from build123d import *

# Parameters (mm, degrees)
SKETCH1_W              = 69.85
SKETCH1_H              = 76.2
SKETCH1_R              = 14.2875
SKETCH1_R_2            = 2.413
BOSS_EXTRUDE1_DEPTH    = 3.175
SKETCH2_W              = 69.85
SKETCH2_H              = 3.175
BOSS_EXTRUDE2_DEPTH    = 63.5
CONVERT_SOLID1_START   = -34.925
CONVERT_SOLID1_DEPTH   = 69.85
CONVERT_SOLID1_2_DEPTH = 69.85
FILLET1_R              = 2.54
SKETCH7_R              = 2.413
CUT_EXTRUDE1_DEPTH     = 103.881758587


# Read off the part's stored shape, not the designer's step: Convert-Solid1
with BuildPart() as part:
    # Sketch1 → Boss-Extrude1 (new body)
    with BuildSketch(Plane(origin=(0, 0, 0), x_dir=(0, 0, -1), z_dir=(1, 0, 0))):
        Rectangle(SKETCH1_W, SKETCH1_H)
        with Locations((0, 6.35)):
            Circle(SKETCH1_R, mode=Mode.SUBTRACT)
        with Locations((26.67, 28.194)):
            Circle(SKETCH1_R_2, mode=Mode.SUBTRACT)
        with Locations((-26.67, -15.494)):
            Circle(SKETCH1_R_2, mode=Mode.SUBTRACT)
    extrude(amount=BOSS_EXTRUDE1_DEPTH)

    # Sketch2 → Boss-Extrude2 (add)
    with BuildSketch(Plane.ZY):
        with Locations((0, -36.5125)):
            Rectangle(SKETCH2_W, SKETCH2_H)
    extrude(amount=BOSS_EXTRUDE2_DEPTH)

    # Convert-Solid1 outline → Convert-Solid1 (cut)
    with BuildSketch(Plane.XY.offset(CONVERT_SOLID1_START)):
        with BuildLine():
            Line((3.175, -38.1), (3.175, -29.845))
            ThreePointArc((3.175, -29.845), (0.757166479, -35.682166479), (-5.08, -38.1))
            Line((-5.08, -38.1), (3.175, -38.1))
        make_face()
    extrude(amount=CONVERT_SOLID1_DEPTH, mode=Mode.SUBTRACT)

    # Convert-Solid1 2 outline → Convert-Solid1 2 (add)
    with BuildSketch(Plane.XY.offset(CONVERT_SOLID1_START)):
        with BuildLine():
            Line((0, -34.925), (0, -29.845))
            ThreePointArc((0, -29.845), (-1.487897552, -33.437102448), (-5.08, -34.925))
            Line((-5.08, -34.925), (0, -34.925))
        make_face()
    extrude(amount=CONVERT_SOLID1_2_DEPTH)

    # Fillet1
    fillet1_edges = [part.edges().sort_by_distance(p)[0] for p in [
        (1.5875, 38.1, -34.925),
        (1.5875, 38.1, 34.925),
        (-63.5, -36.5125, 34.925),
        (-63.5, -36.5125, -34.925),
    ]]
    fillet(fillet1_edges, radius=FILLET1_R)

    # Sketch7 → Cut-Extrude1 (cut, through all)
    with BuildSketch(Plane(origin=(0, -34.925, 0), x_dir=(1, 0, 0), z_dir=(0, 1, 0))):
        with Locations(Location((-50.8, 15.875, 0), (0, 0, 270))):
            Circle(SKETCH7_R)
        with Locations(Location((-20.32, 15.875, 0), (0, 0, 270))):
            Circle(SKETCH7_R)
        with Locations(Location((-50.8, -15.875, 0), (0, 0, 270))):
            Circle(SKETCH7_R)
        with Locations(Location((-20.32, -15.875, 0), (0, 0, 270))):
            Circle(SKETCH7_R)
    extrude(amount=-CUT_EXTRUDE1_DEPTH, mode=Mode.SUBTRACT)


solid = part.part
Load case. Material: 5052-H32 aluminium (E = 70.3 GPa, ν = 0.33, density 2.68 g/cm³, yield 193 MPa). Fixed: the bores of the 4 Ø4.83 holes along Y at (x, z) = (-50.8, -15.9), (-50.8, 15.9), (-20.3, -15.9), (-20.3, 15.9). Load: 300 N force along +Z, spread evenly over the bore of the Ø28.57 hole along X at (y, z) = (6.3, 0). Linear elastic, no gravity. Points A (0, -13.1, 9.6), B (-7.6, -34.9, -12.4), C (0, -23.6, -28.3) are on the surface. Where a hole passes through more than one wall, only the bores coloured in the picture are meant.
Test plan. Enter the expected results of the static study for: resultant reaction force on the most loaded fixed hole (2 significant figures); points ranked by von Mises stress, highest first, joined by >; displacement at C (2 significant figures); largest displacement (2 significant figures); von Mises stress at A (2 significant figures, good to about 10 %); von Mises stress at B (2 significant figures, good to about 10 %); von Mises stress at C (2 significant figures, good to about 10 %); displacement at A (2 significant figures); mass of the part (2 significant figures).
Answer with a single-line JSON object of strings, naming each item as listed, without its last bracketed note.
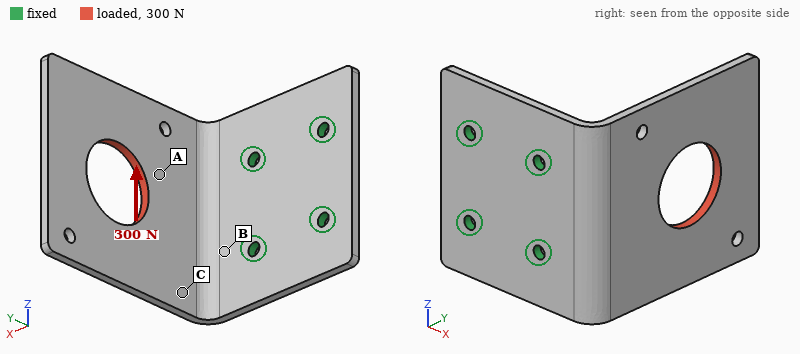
{"resultant reaction force on the most loaded fixed hole": "410 N", "points ranked by von Mises stress, highest first, joined by >": "B > C > A", "displacement at C": "0.15 mm", "largest displacement": "0.40 mm", "von Mises stress at A": "12 MPa", "von Mises stress at B": "41 MPa", "von Mises stress at C": "26 MPa", "displacement at A": "0.12 mm", "mass of the part": "75 g"}
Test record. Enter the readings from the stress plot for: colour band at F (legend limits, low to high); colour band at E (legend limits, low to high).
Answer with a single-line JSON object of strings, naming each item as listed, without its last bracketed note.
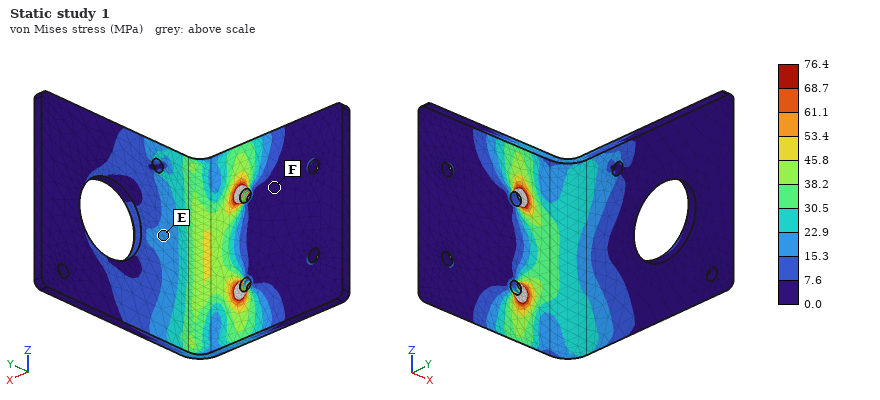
{"colour band at F": "0.0 to 7.6 MPa", "colour band at E": "15.3 to 22.9 MPa"}
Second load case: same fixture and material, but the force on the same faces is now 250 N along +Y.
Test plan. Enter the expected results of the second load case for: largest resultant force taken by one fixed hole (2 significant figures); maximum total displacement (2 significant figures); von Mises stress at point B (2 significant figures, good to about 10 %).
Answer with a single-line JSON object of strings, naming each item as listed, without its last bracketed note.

{"largest resultant force taken by one fixed hole": "150 N", "maximum total displacement": "0.35 mm", "von Mises stress at point B": "18 MPa"}
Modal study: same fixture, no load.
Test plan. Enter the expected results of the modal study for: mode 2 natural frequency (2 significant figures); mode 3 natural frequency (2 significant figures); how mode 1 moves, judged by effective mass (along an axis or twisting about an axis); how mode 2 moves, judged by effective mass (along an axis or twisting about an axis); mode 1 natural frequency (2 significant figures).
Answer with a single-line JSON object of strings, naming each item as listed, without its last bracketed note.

{"mode 2 natural frequency": "810 Hz", "mode 3 natural frequency": "1200 Hz", "how mode 1 moves, judged by effective mass": "along X", "how mode 2 moves, judged by effective mass": "along Z", "mode 1 natural frequency": "350 Hz"}
